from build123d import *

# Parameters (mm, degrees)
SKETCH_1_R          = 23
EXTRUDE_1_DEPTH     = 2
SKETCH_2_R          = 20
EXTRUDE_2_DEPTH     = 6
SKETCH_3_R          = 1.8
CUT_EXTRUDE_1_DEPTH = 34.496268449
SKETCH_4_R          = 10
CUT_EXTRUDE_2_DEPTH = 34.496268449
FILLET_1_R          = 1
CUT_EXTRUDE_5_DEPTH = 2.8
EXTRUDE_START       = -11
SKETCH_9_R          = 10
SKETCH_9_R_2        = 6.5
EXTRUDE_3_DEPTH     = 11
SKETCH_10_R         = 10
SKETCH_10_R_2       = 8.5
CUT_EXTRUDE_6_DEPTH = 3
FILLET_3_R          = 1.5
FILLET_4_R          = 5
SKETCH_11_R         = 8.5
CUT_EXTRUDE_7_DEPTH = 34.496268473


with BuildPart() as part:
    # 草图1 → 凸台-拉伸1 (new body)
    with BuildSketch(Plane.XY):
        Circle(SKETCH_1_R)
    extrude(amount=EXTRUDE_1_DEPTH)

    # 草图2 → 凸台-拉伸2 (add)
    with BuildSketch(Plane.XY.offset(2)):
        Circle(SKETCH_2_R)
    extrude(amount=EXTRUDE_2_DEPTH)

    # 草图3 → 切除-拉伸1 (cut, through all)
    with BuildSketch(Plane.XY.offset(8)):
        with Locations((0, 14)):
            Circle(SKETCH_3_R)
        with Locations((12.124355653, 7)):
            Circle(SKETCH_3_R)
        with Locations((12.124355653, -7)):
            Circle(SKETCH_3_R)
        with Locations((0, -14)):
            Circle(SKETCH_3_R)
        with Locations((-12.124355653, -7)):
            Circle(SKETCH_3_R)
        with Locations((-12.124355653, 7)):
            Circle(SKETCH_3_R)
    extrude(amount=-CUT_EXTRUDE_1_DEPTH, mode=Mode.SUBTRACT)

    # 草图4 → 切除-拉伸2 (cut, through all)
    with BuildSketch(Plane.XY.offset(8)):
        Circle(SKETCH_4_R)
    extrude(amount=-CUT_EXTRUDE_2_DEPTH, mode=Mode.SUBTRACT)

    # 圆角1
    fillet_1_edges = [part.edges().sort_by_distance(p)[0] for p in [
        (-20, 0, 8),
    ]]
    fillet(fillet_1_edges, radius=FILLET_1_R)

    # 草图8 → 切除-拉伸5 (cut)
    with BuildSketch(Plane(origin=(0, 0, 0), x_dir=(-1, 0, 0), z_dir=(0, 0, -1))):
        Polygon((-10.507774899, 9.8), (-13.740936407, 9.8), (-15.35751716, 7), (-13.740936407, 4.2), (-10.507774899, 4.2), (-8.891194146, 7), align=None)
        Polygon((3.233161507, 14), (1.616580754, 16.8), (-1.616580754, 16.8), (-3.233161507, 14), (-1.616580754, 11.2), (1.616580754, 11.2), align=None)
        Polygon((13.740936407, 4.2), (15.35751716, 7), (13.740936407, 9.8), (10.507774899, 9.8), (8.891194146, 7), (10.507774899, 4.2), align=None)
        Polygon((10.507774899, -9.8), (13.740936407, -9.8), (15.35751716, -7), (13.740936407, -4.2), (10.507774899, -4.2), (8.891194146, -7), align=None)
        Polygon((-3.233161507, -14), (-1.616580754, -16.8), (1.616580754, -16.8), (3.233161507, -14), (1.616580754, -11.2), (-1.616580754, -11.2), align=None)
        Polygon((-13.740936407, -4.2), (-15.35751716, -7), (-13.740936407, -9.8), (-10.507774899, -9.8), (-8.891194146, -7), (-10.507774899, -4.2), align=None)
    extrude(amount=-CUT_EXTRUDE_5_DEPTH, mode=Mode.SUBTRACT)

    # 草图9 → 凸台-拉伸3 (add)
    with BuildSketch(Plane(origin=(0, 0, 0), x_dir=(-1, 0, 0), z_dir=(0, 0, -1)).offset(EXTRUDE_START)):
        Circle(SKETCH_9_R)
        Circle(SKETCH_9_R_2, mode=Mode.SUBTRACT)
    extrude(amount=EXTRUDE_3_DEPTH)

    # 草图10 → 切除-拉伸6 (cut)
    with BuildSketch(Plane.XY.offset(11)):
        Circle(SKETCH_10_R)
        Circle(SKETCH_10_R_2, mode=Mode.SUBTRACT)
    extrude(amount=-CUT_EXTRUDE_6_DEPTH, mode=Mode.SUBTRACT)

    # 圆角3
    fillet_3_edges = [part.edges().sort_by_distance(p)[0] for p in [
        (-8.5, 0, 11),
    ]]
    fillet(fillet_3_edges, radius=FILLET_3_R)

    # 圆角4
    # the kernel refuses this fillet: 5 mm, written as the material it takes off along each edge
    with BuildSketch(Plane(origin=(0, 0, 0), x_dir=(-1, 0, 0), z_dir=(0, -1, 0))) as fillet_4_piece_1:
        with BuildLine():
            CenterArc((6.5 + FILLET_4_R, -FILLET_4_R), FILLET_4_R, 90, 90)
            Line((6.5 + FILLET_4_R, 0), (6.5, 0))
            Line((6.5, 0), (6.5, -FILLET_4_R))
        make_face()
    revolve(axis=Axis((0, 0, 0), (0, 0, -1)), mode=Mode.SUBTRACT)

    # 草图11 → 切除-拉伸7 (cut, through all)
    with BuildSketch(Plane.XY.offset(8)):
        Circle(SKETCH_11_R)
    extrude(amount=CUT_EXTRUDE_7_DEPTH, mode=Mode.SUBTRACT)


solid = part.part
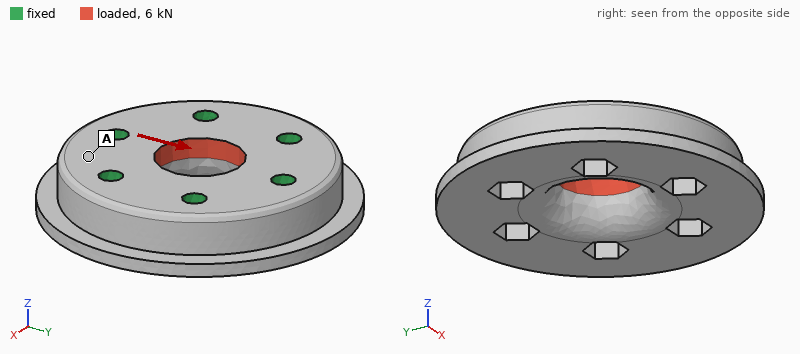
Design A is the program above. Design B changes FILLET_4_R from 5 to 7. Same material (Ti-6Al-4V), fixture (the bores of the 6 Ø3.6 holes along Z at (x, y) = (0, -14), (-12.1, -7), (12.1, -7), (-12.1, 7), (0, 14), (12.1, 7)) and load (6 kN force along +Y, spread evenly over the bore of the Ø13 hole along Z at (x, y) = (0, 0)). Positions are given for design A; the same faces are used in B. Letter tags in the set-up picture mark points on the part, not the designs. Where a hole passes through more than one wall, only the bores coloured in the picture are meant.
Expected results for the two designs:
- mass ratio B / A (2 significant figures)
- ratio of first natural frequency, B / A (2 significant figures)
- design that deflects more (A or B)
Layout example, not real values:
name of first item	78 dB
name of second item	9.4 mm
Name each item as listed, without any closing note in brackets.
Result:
mass ratio B / A	0.97
ratio of first natural frequency, B / A	0.99
design that deflects more	B
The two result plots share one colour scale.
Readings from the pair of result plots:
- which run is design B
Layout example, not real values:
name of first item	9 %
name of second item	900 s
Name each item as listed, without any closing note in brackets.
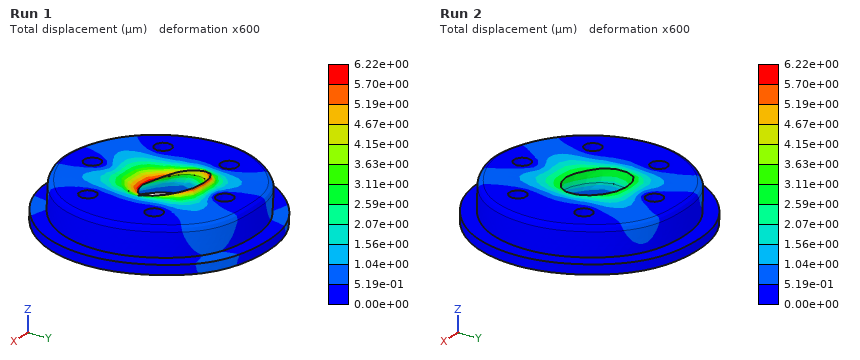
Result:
which run is design B	Run 1
